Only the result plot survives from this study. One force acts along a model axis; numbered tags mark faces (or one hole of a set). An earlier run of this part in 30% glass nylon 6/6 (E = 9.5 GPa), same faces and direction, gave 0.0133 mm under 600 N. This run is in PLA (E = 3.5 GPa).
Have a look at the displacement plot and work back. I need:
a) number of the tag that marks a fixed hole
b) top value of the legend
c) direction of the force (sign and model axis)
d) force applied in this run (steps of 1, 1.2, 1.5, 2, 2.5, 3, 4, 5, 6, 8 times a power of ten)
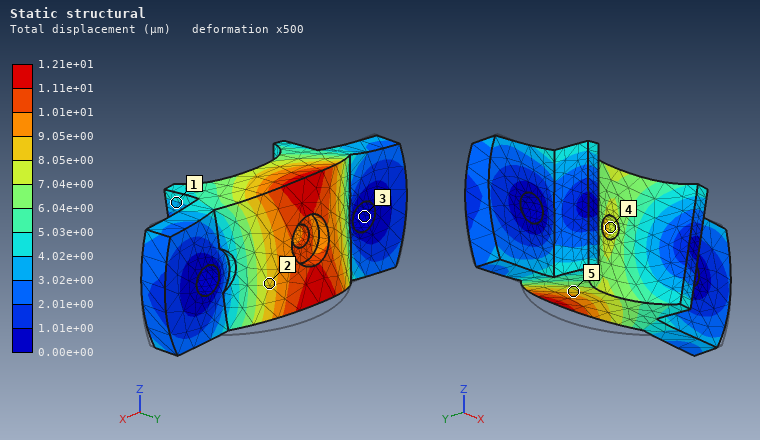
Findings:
3
1.21e+01 µm
+Z
200 N
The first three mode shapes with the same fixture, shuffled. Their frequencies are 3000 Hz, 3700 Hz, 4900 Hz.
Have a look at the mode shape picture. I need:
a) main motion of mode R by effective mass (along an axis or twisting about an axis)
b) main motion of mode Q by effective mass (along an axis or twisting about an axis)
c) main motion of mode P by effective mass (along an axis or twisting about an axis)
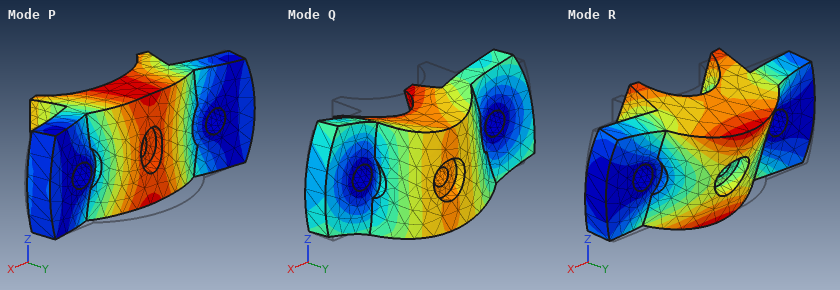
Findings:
twisting about X
along Z
along Y
